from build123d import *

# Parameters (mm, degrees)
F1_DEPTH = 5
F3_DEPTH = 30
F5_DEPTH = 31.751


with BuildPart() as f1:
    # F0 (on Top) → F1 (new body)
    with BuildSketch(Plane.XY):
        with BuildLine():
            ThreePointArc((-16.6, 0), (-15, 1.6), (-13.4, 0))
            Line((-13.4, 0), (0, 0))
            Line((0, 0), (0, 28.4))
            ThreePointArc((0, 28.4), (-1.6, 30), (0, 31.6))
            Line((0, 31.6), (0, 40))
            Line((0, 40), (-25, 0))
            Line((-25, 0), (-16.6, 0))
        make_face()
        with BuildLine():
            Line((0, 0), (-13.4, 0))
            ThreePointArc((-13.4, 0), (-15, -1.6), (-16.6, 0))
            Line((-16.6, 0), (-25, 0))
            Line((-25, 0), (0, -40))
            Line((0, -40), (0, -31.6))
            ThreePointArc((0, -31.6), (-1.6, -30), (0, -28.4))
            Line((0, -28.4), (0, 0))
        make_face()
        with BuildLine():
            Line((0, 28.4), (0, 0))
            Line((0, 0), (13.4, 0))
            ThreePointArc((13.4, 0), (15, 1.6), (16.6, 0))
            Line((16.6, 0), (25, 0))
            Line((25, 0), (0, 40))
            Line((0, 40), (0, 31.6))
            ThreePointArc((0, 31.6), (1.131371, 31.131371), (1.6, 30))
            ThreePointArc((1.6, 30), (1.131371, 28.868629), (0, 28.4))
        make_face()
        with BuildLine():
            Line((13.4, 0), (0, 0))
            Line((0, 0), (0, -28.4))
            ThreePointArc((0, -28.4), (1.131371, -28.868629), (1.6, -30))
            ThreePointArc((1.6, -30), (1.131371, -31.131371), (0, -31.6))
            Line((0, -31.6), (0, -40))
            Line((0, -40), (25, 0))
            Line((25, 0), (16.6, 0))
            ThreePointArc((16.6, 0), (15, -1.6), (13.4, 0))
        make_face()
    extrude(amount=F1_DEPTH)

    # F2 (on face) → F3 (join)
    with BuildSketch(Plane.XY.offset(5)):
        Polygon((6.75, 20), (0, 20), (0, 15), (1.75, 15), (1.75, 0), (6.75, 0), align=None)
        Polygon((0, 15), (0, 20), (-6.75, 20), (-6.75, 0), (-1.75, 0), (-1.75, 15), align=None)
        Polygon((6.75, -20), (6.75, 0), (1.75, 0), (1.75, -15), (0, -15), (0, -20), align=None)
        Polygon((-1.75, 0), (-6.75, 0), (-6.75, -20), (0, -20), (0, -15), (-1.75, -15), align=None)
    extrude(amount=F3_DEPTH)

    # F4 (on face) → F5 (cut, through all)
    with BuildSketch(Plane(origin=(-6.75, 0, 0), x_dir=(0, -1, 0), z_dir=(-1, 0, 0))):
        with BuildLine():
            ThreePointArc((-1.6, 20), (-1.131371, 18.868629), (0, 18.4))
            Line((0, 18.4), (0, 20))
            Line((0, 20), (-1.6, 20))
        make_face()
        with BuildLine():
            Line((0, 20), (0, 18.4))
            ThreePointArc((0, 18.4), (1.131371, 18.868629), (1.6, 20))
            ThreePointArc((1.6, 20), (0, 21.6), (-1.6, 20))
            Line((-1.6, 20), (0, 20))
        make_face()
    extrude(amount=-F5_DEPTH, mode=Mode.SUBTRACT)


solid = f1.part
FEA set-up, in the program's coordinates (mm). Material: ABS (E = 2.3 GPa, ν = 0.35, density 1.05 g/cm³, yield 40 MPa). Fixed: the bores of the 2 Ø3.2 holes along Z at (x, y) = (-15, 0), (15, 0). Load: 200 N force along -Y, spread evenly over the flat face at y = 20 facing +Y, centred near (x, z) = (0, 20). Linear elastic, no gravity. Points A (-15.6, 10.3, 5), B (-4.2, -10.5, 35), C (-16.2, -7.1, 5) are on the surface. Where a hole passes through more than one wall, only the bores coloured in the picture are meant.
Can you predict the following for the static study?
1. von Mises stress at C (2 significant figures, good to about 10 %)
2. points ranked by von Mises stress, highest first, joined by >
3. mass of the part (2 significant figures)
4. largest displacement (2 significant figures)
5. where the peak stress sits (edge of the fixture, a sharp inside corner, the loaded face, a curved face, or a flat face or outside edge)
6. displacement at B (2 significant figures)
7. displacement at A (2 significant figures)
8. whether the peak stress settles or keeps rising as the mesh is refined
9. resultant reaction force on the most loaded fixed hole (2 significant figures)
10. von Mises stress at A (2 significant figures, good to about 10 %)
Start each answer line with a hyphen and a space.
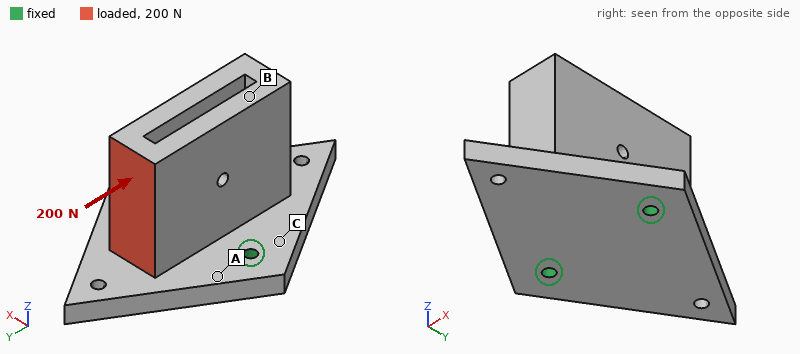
- 8.3 MPa
- C > A > B
- 24 g
- 0.80 mm
- edge of the fixture
- 0.65 mm
- 0.14 mm
- keeps rising
- 100 N
- 5.9 MPa
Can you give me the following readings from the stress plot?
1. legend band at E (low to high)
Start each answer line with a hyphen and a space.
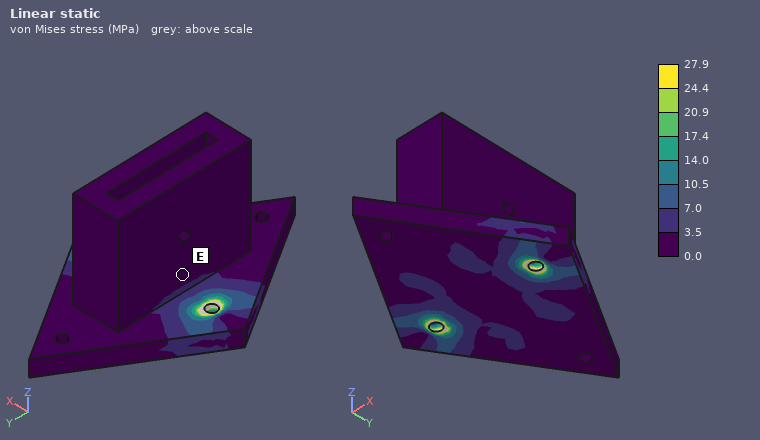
- 0.0 to 3.5 MPa
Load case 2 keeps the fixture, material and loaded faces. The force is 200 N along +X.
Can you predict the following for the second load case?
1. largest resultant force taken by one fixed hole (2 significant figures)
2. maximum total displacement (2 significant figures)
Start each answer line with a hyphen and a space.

- 210 N
- 0.33 mm
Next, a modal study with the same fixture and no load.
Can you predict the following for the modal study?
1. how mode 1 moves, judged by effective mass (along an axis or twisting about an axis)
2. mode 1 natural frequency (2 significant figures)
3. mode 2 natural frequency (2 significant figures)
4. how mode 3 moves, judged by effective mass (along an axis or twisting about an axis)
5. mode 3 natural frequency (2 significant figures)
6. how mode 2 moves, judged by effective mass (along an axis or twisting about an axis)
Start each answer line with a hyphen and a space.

- along Y
- 690 Hz
- 1500 Hz
- along Z
- 2200 Hz
- along X
